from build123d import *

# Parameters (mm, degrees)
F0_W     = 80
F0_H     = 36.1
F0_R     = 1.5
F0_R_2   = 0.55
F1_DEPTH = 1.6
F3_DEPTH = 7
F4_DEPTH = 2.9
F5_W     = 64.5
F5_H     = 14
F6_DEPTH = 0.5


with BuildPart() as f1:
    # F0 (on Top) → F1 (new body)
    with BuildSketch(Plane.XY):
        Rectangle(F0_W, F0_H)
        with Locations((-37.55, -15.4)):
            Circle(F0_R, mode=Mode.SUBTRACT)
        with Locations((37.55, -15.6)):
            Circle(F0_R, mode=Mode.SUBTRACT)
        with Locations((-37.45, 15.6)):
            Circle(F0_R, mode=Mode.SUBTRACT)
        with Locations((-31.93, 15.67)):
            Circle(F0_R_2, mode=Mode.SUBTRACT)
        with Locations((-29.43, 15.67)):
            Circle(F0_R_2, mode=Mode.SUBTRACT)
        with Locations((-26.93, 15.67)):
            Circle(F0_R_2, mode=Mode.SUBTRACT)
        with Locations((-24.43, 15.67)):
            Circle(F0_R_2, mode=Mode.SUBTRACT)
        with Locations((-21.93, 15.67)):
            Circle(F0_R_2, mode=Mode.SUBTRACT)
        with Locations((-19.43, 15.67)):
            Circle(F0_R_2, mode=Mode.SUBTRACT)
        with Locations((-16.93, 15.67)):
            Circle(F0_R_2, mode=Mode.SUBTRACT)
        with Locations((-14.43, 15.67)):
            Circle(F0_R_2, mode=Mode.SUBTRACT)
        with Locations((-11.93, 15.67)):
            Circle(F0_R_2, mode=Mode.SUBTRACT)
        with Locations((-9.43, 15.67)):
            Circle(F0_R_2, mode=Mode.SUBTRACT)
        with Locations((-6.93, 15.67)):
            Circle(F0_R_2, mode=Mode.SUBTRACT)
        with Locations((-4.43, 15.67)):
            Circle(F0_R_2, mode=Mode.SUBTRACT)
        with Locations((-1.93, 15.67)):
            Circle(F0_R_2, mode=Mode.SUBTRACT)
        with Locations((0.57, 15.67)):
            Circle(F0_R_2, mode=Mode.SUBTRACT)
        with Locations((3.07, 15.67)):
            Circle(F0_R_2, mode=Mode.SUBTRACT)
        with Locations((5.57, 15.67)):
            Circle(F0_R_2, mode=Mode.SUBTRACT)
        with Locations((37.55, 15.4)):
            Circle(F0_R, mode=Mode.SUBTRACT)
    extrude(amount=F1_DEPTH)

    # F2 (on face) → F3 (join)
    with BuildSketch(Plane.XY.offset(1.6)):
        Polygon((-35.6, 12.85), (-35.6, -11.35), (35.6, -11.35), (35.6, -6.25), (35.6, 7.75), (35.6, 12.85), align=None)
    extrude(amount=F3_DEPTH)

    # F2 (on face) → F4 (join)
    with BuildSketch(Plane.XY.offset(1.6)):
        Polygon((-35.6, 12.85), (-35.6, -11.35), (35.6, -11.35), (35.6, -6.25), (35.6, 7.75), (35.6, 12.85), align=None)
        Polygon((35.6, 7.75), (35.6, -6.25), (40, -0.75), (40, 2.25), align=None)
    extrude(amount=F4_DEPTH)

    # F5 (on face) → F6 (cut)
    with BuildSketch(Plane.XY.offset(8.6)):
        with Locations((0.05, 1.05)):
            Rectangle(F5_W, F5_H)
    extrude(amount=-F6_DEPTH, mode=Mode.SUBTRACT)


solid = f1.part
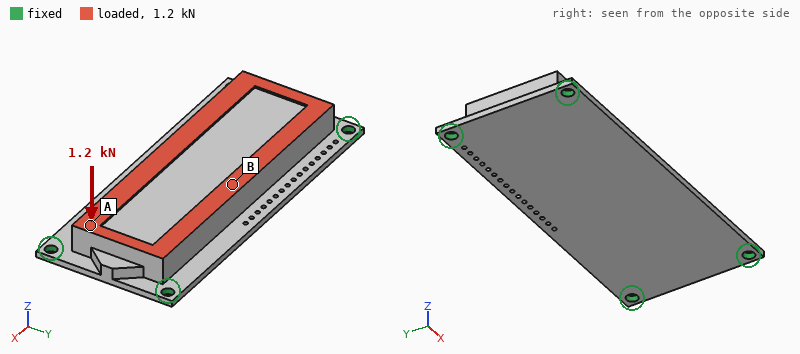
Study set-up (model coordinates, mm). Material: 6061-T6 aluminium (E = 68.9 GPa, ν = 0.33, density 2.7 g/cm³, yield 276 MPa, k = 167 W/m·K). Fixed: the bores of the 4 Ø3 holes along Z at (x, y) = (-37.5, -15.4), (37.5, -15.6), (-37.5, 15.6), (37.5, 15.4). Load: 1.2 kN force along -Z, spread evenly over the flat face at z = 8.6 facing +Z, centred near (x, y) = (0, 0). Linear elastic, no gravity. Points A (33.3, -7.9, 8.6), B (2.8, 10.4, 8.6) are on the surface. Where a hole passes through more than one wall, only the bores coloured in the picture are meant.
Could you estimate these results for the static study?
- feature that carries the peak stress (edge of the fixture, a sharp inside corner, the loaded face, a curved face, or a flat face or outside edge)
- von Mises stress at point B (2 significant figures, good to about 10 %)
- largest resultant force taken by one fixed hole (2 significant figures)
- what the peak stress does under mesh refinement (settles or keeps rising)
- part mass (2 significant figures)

edge of the fixture
28 MPa
560 N
keeps rising
44 g
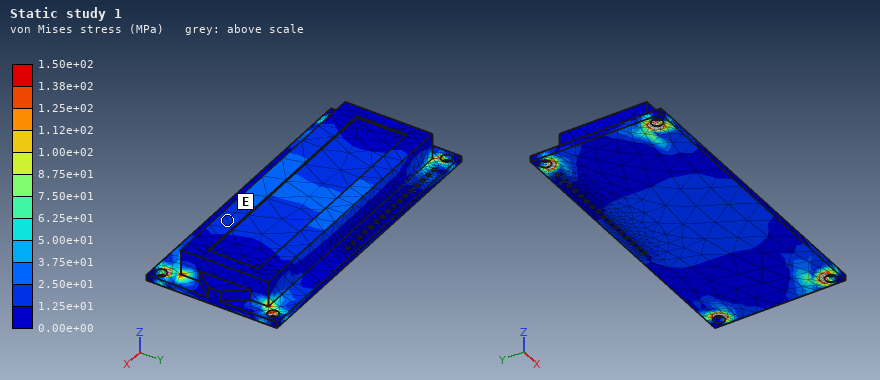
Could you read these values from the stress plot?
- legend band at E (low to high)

1.25e+01 to 2.50e+01 MPa
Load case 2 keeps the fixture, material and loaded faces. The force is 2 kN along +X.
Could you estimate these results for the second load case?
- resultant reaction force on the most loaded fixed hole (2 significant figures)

590 N
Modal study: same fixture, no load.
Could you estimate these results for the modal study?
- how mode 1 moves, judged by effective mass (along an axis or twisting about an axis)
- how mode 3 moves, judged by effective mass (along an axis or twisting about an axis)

along Z
twisting about Y
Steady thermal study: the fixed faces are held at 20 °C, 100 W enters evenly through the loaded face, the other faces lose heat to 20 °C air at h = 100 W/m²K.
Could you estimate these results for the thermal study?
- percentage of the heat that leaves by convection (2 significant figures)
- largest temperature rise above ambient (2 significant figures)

30 %
57 K
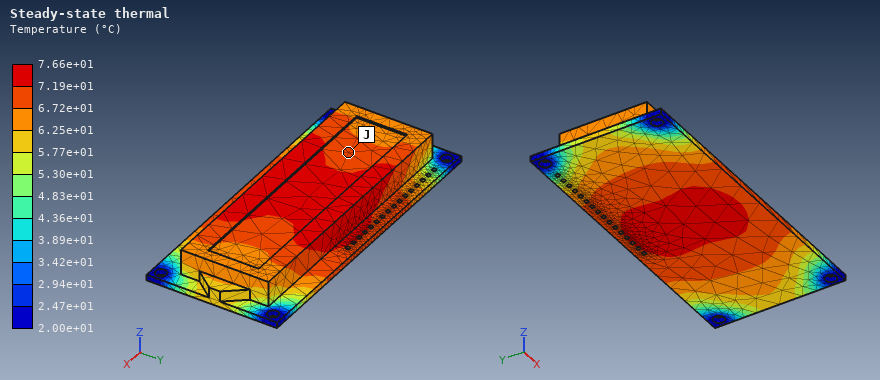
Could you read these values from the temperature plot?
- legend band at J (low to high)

6.72e+01 to 7.19e+01 °C
